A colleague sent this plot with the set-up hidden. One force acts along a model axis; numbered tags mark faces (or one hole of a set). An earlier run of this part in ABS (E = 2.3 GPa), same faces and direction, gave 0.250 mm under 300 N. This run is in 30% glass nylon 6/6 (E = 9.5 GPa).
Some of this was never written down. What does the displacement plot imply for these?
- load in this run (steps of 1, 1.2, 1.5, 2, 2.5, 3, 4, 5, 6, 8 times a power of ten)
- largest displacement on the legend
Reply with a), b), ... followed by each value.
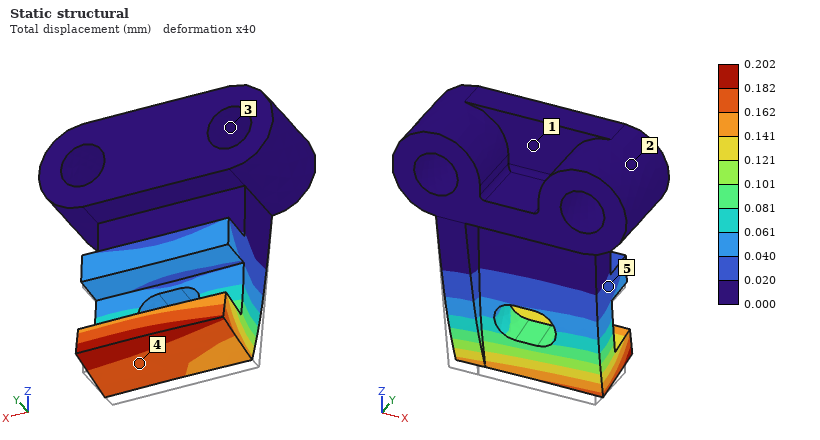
a) 1 kN
b) 0.202 mm
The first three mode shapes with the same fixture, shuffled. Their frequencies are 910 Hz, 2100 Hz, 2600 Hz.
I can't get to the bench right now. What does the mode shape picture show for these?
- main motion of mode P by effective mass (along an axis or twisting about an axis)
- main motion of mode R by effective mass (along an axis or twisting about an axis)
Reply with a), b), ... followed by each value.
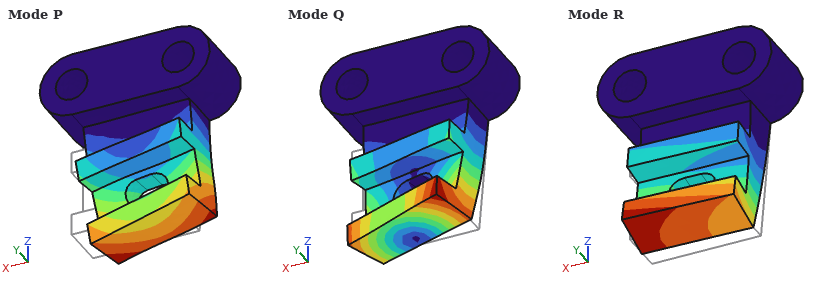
a) along X
b) along Y
